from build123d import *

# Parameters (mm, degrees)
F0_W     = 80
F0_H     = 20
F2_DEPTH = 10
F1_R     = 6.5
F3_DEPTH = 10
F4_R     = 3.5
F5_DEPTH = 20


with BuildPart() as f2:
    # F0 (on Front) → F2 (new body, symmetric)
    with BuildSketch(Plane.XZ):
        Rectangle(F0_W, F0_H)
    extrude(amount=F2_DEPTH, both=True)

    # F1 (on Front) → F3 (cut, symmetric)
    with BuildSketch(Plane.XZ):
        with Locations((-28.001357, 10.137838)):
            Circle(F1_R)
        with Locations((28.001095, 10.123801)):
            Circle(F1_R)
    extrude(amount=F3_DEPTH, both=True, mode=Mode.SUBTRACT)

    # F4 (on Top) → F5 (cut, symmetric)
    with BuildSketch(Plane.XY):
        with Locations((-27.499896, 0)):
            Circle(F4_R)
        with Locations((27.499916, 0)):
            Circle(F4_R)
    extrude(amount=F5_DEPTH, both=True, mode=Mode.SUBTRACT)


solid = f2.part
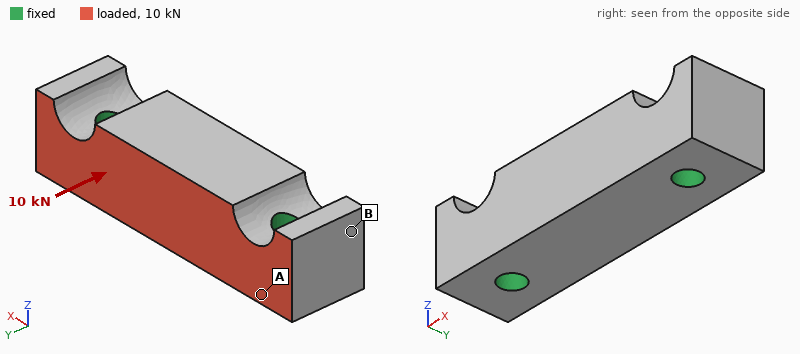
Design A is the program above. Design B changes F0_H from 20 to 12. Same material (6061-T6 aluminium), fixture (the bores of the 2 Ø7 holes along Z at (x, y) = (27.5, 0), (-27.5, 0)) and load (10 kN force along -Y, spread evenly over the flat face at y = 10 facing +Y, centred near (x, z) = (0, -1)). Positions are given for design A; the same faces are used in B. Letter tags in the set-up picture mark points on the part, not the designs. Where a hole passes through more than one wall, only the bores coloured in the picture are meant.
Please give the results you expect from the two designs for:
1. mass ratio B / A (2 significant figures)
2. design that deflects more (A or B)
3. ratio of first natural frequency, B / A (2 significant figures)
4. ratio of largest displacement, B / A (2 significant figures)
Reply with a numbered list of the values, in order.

1. 0.63
2. B
3. 0.94
4. 1.2
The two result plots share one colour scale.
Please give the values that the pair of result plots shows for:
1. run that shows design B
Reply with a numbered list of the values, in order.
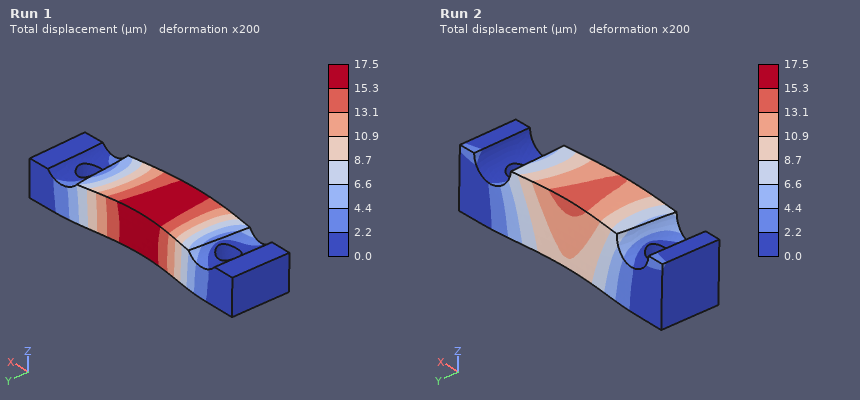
1. Run 1
